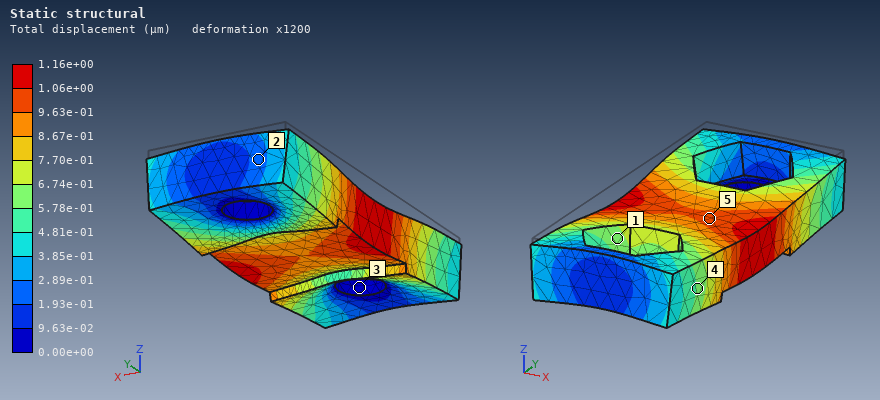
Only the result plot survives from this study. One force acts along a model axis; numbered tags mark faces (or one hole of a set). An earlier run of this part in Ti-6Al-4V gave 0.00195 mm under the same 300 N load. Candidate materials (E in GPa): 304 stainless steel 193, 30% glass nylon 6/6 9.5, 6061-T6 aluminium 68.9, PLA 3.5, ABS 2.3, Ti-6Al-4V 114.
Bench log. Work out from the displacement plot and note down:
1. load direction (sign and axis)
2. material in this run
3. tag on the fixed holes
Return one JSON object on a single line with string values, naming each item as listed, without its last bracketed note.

{"load direction": "-Z", "material in this run": "304 stainless steel", "tag on the fixed holes": "3"}
